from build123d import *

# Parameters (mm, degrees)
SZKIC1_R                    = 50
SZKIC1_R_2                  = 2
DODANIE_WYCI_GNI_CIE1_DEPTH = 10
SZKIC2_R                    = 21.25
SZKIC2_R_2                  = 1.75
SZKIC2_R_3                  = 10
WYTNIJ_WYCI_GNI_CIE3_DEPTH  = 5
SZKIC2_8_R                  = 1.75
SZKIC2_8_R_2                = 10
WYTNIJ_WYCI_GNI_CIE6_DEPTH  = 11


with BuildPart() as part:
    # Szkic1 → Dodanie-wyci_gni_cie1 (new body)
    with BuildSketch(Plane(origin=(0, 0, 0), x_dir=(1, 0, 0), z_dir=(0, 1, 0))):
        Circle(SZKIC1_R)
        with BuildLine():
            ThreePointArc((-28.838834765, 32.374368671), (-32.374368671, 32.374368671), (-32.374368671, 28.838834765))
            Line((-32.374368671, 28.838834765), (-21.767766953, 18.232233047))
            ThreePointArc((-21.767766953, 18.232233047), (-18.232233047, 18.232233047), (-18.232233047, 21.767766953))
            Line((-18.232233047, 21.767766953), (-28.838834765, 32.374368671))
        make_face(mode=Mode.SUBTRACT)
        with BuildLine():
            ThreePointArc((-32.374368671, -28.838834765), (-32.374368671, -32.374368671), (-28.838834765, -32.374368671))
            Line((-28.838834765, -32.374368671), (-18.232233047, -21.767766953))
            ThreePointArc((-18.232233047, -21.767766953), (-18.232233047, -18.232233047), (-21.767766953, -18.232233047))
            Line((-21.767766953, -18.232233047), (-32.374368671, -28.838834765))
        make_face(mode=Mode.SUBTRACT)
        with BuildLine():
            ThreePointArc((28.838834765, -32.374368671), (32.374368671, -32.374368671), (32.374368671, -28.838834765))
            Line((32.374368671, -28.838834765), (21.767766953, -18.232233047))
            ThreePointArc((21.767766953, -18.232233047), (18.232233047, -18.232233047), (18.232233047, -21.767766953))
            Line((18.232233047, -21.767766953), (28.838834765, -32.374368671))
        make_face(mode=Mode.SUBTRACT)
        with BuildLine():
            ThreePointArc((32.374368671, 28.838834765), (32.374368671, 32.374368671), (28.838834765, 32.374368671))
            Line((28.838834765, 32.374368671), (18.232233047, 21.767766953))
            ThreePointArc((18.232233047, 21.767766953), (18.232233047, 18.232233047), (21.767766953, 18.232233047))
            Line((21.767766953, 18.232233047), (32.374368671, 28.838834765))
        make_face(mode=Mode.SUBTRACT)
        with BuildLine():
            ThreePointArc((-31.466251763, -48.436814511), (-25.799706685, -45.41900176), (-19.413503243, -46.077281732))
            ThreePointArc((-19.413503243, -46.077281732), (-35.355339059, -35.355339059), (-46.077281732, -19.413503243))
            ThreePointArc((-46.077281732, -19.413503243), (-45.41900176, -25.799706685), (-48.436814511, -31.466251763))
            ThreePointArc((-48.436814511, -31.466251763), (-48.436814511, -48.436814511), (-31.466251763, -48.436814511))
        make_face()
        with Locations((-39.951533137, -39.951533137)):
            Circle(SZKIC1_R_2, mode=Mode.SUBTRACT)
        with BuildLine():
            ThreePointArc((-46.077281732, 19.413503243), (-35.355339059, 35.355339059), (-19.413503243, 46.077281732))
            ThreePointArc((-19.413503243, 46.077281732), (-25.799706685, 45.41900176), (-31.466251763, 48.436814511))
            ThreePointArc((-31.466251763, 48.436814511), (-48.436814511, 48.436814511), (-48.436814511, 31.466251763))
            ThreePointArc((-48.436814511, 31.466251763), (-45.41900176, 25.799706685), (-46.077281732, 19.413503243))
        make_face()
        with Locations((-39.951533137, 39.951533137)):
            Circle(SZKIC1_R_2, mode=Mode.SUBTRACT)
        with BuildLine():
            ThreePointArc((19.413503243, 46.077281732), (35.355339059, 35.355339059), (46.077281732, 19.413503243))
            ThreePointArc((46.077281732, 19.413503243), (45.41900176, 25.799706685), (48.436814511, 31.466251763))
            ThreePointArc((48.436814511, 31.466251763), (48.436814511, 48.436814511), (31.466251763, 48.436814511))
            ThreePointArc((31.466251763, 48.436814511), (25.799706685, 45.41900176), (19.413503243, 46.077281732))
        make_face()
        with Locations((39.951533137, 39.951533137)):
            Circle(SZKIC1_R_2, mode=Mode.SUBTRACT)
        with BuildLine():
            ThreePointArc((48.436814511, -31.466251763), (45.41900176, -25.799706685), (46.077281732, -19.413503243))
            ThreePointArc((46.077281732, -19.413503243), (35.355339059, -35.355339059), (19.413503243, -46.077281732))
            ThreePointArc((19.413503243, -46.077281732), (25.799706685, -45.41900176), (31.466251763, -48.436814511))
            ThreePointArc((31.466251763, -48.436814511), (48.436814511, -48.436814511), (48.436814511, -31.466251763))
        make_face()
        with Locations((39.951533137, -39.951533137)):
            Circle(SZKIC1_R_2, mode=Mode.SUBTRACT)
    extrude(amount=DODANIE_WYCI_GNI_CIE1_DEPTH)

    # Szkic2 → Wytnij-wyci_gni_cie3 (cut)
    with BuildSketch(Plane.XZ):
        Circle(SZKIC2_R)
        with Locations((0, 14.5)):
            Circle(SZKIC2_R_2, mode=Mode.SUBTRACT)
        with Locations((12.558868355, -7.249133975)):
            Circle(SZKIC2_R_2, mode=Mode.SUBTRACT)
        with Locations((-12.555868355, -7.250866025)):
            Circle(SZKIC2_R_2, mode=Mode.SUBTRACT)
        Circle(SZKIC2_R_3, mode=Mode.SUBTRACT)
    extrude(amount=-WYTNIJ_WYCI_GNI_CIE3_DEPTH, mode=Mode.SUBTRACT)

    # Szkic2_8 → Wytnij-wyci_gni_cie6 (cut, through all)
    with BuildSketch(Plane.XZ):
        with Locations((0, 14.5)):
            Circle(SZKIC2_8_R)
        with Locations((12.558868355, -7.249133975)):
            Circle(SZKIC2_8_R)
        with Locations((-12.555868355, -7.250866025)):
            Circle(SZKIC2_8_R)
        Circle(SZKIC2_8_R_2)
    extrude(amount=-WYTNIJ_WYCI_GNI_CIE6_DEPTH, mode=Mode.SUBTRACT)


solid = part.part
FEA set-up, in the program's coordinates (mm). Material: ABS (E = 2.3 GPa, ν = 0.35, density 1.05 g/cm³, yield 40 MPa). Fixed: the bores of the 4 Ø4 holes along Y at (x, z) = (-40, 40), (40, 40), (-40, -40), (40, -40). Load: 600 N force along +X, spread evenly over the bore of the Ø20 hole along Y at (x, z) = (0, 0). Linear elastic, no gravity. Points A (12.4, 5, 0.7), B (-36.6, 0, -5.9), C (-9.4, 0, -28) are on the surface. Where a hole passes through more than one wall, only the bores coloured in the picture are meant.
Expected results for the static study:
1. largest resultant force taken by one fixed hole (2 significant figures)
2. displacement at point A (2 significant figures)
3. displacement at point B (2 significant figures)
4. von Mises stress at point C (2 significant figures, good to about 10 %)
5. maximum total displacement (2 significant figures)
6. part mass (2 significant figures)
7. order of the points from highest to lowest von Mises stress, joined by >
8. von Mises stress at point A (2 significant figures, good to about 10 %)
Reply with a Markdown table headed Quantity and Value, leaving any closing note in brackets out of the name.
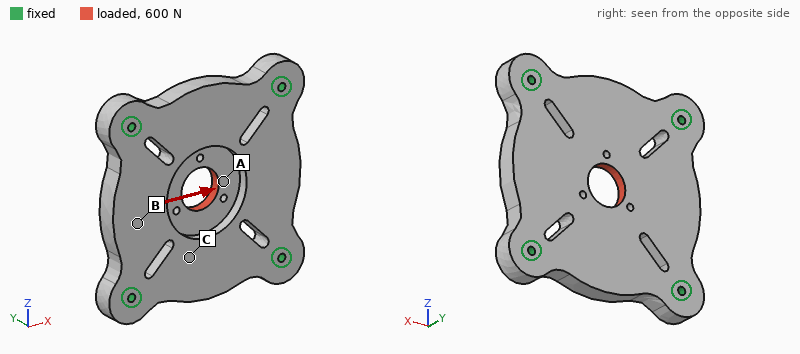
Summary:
| Quantity | Value |
|---|---|
| largest resultant force taken by one fixed hole | 170 N |
| displacement at point A | 32 µm |
| displacement at point B | 20 µm |
| von Mises stress at point C | 0.72 MPa |
| maximum total displacement | 37 µm |
| part mass | 86 g |
| order of the points from highest to lowest von Mises stress, joined by > | A > C > B |
| von Mises stress at point A | 1.8 MPa |
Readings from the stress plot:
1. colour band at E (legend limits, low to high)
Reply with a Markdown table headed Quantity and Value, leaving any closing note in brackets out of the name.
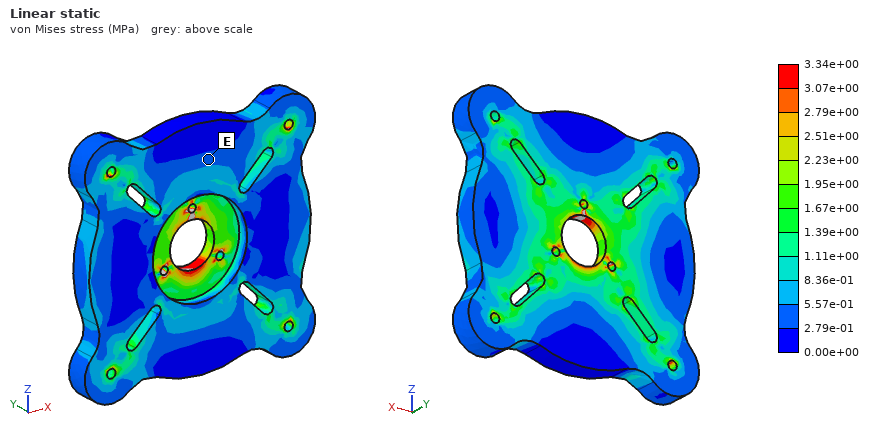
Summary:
| Quantity | Value |
|---|---|
| colour band at E | 2.79e-01 to 5.57e-01 MPa |
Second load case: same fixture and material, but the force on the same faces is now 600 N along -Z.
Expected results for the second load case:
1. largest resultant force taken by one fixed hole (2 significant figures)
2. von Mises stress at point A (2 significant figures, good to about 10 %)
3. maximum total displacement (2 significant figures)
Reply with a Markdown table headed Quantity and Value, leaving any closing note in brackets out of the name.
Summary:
| Quantity | Value |
|---|---|
| largest resultant force taken by one fixed hole | 170 N |
| von Mises stress at point A | 2.9 MPa |
| maximum total displacement | 39 µm |
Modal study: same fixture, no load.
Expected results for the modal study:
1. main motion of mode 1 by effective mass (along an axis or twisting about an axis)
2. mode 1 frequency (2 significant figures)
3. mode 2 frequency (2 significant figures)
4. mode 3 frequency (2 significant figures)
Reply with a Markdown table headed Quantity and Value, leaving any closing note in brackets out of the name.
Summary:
| Quantity | Value |
|---|---|
| main motion of mode 1 by effective mass | along Y |
| mode 1 frequency | 1400 Hz |
| mode 2 frequency | 2100 Hz |
| mode 3 frequency | 2100 Hz |
